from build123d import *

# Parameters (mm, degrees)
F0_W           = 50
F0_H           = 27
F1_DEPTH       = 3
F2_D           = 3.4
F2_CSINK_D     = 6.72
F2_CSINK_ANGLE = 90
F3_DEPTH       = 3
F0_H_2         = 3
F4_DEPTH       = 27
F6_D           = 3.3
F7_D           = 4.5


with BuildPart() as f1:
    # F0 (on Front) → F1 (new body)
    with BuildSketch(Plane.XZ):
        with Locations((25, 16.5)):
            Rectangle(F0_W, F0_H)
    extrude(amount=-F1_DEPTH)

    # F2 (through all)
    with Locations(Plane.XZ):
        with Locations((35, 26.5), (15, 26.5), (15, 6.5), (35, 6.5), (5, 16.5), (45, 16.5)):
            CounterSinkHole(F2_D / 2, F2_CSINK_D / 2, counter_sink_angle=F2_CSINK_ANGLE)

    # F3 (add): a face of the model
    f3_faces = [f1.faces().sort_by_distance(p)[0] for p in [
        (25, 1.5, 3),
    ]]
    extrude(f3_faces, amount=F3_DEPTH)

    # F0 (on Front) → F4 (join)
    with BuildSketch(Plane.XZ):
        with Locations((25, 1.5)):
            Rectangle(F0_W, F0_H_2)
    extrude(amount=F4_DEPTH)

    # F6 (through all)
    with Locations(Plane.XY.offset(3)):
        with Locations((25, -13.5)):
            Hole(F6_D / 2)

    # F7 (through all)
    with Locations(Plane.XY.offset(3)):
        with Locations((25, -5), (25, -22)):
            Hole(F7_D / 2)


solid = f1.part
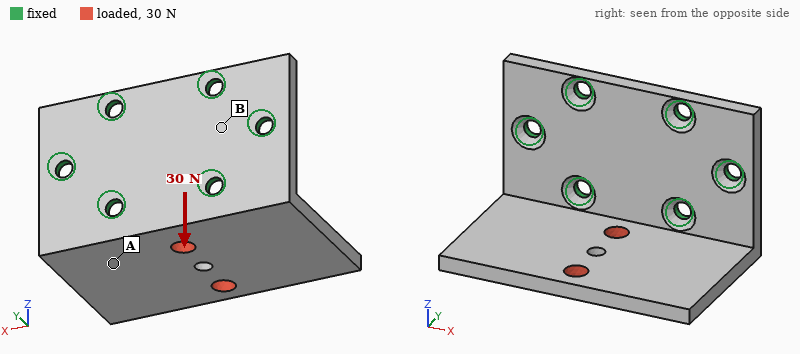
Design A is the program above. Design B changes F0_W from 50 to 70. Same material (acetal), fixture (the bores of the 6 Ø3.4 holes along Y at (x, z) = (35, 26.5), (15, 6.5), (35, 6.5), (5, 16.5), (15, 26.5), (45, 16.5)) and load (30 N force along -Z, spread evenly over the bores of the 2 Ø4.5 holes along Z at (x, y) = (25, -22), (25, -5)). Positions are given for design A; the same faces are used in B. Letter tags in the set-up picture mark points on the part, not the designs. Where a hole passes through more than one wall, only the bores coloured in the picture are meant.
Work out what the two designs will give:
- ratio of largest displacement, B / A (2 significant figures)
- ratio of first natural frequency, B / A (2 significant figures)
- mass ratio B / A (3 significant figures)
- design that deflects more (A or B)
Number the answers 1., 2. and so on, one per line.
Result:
1. 0.81
2. 0.98
3. 1.42
4. A
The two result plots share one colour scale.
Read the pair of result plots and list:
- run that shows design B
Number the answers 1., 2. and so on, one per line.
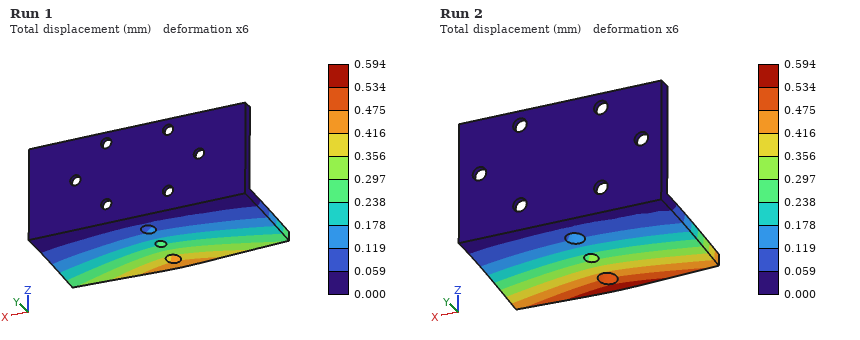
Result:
1. Run 1
